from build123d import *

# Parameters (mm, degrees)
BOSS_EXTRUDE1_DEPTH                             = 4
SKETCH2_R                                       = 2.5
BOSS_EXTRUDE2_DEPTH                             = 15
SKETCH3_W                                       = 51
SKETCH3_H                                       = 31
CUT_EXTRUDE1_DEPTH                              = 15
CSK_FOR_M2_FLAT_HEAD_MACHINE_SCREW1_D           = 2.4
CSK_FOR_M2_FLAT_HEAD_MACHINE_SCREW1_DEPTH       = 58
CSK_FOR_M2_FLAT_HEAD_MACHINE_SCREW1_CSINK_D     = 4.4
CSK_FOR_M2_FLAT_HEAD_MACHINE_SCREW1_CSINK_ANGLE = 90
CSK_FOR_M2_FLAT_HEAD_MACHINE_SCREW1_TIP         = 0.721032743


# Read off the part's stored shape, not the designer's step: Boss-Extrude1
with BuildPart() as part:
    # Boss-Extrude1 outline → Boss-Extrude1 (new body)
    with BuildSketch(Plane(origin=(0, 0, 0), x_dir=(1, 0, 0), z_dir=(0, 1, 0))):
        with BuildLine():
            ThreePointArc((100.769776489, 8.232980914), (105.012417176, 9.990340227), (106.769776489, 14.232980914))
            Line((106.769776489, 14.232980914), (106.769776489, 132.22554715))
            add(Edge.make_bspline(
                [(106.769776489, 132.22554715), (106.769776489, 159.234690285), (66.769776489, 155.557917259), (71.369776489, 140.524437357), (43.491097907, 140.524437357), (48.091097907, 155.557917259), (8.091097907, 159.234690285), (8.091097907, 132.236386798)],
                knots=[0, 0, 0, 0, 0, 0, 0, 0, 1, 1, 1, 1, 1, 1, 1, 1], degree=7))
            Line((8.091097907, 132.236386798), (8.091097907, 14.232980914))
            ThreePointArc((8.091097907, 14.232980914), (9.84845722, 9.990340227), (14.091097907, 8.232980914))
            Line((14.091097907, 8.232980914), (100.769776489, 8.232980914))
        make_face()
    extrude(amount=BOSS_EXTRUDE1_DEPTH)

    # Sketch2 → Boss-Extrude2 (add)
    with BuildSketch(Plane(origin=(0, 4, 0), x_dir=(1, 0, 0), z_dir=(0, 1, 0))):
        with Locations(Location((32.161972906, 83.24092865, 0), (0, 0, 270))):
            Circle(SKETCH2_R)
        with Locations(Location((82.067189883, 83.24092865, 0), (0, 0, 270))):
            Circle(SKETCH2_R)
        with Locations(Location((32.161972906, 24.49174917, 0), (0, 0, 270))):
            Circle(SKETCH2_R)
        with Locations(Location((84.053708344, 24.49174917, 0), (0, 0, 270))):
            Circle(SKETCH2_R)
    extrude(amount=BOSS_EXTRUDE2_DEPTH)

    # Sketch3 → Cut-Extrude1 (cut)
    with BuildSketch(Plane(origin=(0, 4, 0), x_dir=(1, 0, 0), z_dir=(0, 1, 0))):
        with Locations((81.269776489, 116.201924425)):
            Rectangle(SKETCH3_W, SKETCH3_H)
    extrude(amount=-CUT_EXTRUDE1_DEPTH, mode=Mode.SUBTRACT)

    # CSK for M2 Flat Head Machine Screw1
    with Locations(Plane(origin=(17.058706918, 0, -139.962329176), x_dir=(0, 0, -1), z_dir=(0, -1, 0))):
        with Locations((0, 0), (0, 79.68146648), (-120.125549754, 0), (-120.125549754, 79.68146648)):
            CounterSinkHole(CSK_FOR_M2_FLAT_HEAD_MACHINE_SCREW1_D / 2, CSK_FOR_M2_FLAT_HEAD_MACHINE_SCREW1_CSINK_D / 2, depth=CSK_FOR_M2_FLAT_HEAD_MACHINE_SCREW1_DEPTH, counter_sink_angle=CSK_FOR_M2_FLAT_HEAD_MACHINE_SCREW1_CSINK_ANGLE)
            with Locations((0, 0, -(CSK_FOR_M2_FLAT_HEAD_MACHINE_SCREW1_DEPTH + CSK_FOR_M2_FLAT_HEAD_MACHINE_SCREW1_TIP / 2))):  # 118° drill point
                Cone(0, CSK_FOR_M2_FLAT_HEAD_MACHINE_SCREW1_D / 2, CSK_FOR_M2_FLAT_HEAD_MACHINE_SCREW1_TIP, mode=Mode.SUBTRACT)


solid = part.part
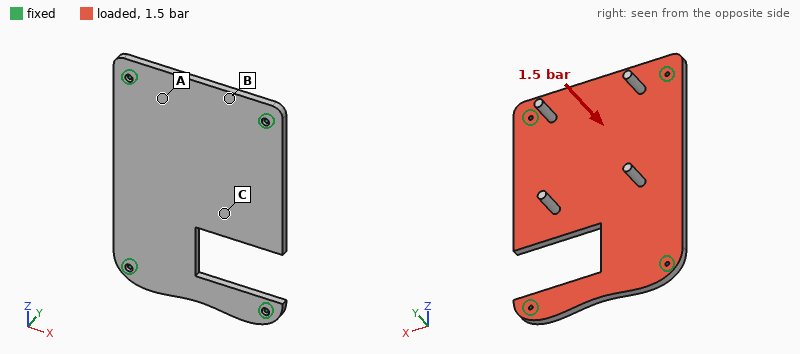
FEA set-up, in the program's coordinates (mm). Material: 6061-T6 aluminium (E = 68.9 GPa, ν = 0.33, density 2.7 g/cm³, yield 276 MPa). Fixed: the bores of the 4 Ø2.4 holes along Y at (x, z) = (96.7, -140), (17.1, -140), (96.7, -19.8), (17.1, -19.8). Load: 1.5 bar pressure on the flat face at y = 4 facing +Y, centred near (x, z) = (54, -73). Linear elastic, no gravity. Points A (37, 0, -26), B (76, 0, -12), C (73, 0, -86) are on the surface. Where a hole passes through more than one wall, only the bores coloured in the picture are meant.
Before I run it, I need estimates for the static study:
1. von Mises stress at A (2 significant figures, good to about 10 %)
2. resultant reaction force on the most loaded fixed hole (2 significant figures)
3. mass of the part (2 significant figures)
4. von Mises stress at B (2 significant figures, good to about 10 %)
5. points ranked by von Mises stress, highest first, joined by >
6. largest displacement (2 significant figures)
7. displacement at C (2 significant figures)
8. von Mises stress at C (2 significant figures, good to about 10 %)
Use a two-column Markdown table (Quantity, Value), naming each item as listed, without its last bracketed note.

| Quantity | Value |
|---|---|
| von Mises stress at A | 26 MPa |
| resultant reaction force on the most loaded fixed hole | 650 N |
| mass of the part | 130 g |
| von Mises stress at B | 15 MPa |
| points ranked by von Mises stress, highest first, joined by > | C > A > B |
| largest displacement | 1.2 mm |
| displacement at C | 0.78 mm |
| von Mises stress at C | 53 MPa |
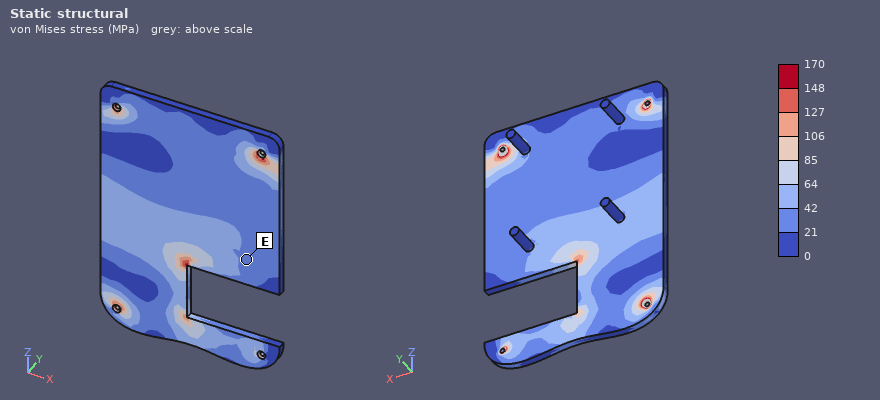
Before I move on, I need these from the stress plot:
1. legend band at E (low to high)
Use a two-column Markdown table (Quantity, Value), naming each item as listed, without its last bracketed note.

| Quantity | Value |
|---|---|
| legend band at E | 21 to 42 MPa |
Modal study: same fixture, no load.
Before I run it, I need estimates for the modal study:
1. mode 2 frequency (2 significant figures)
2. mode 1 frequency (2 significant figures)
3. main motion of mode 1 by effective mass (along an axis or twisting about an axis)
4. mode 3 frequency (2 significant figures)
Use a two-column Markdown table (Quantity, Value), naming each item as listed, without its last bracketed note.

| Quantity | Value |
|---|---|
| mode 2 frequency | 1400 Hz |
| mode 1 frequency | 760 Hz |
| main motion of mode 1 by effective mass | along Y |
| mode 3 frequency | 2400 Hz |
